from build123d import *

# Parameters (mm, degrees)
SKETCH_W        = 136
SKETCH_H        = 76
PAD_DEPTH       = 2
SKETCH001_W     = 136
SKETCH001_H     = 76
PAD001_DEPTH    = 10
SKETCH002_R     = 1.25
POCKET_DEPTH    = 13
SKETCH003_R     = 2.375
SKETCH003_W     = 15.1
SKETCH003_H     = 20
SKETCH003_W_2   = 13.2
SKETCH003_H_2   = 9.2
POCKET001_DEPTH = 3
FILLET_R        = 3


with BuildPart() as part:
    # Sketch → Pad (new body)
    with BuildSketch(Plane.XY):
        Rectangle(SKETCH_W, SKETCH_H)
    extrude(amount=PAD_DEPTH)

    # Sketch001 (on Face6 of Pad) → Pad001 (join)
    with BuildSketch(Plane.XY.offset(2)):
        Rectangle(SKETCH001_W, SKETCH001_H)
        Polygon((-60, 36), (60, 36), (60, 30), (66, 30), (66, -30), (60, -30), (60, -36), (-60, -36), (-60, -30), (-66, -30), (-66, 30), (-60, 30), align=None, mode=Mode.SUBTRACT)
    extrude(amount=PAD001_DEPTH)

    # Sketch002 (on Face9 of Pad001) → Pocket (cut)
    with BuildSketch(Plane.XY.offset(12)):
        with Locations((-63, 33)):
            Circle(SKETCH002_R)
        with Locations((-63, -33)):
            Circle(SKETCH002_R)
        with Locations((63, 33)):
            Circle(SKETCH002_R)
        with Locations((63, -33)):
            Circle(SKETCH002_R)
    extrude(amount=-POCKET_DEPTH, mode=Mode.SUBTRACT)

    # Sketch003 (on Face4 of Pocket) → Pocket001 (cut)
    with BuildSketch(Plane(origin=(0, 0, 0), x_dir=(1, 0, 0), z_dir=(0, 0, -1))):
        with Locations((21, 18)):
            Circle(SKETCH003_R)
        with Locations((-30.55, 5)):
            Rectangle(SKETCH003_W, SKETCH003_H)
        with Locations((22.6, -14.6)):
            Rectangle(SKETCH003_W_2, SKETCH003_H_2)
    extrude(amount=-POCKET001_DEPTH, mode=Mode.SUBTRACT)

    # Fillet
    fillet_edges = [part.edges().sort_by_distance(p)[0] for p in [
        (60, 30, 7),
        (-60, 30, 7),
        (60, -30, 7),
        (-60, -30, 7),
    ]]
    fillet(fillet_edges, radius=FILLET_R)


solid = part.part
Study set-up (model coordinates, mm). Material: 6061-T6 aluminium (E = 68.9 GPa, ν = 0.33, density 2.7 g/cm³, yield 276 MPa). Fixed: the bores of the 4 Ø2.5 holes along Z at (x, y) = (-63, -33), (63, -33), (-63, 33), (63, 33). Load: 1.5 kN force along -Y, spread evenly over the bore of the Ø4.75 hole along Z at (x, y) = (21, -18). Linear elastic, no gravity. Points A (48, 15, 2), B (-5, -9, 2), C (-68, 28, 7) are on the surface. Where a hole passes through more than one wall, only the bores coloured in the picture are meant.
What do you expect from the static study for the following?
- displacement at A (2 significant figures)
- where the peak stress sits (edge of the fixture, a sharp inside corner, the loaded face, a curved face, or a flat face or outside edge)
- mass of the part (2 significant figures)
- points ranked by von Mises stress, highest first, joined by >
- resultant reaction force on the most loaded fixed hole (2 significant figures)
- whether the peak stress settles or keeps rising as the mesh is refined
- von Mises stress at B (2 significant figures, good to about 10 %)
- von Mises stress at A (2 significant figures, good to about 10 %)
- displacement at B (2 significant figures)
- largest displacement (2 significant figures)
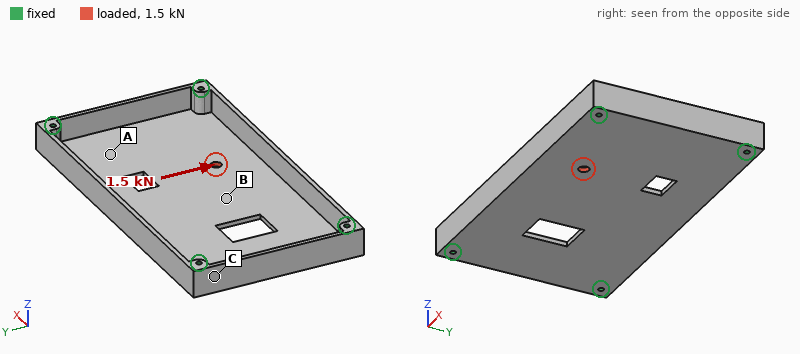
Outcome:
7.2 µm
a sharp inside corner
79 g
A > B > C
670 N
keeps rising
9.5 MPa
17 MPa
15 µm
30 µm
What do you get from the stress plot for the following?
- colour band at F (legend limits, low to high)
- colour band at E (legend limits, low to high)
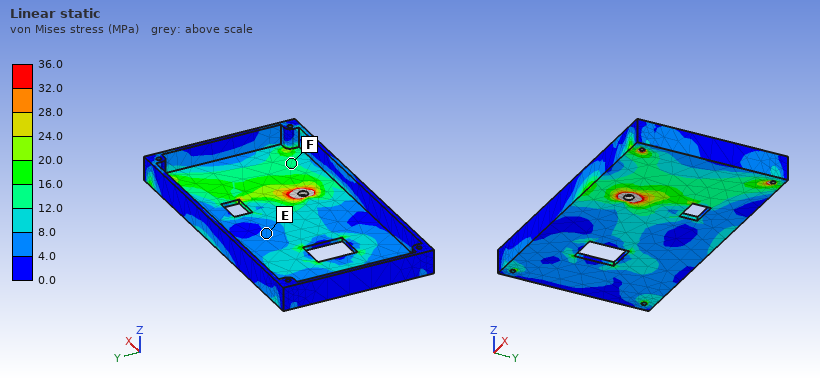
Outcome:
12.0 to 16.0 MPa
4.0 to 8.0 MPa
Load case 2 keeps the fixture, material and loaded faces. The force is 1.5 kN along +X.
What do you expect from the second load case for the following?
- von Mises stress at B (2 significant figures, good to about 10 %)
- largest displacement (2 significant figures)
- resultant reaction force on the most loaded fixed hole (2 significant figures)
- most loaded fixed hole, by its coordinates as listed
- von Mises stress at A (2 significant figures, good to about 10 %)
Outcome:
5.8 MPa
13 µm
660 N
(63, -33)
6.5 MPa
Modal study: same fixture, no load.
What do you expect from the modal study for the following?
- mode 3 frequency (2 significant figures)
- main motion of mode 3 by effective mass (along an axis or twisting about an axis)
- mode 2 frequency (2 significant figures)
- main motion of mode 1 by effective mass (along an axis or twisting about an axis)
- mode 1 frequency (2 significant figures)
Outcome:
2800 Hz
twisting about X
2300 Hz
along Z
1200 Hz
